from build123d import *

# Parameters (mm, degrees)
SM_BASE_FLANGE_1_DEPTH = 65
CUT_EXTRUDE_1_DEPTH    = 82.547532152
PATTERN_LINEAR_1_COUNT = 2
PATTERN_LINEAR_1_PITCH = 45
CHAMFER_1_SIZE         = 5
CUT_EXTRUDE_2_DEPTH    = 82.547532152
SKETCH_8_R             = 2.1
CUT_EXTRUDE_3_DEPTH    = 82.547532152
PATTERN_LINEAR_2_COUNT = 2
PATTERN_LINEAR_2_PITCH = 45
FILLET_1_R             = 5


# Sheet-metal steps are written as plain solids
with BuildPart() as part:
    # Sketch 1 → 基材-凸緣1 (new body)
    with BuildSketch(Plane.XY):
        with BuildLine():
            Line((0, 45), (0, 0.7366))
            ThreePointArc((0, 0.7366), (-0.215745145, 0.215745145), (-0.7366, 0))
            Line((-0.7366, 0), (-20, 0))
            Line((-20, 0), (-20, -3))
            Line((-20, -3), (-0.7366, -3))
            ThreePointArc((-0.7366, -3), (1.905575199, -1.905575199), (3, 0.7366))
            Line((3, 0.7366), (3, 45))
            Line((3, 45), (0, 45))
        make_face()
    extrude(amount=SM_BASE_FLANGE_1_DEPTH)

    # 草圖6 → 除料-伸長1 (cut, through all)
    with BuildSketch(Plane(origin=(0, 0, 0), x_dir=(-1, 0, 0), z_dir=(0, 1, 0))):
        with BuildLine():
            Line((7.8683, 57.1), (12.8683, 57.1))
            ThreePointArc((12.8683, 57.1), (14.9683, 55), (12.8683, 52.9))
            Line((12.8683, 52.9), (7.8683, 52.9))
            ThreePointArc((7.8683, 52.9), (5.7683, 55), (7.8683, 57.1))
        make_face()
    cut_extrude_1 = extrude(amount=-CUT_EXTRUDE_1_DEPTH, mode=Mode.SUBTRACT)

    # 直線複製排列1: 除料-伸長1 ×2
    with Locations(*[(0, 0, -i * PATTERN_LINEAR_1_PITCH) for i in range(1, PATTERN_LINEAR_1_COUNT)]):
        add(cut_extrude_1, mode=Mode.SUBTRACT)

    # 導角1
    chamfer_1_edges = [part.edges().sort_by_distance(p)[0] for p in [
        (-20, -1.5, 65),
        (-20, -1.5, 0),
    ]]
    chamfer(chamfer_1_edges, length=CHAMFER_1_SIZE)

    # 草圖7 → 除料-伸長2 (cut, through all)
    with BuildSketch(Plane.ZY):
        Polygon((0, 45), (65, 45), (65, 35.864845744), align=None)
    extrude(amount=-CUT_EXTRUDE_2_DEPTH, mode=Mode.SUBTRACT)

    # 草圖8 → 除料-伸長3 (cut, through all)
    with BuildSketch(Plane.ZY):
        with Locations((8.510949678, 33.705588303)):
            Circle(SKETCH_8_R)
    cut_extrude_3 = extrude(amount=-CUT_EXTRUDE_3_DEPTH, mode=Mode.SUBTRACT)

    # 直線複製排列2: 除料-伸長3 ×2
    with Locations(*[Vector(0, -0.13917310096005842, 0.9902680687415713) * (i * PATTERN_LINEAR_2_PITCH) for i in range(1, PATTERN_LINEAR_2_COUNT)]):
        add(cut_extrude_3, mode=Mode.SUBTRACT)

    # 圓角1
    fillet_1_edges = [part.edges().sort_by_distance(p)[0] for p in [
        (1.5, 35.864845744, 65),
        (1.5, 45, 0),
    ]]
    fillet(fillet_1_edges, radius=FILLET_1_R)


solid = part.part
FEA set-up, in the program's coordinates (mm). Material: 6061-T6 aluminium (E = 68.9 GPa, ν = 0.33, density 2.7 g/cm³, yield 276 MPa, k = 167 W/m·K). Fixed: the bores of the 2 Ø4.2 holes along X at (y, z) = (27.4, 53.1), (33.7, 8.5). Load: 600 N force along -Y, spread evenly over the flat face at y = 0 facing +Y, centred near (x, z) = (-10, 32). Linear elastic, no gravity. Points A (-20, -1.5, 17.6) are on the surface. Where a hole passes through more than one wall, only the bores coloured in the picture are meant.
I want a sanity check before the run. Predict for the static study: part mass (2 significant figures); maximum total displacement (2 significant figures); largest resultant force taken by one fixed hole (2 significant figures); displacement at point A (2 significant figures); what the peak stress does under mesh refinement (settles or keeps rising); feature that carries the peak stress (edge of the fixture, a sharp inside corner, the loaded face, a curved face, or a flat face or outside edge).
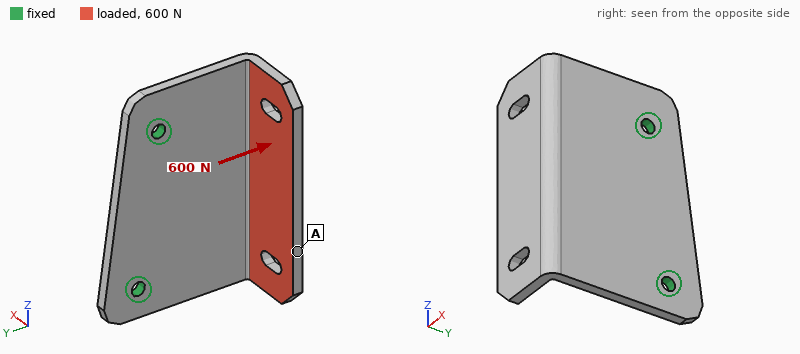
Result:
32 g
0.70 mm
320 N
0.66 mm
keeps rising
edge of the fixture
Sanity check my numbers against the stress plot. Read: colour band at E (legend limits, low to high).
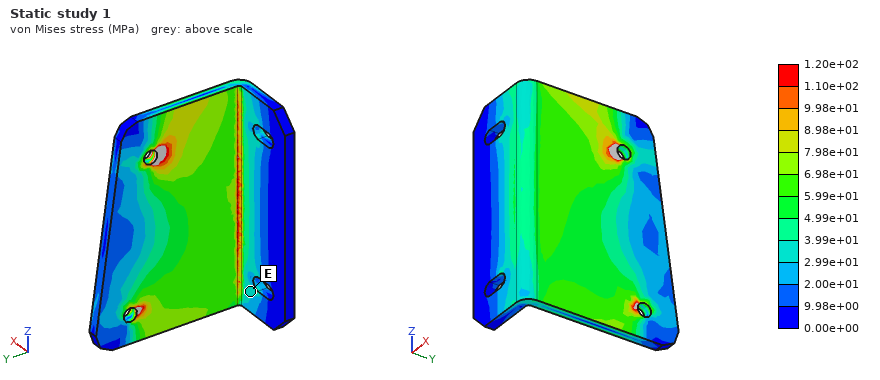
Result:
2.99e+01 to 3.99e+01 MPa
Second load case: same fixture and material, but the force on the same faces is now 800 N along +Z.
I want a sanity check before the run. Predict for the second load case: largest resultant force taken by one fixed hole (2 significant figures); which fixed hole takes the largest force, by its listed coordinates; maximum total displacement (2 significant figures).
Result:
730 N
(27.4, 53.1)
0.42 mm
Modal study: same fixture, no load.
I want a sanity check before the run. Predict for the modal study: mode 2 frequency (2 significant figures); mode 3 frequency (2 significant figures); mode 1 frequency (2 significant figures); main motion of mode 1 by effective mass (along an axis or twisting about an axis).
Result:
2000 Hz
3700 Hz
1100 Hz
along X
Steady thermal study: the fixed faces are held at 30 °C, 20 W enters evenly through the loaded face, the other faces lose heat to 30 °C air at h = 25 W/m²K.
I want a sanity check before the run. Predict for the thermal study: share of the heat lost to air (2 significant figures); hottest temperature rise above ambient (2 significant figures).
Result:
13 %
28 K
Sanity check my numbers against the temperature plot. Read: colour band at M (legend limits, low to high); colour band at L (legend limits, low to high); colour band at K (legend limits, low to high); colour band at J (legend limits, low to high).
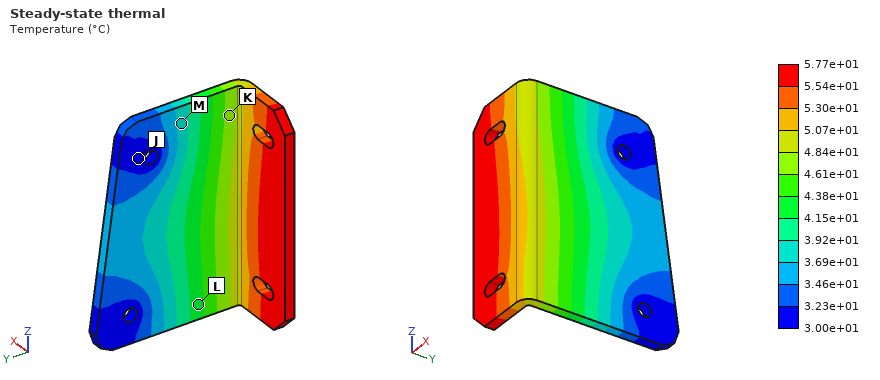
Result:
3.69e+01 to 3.92e+01 °C
4.15e+01 to 4.38e+01 °C
4.61e+01 to 4.84e+01 °C
3.00e+01 to 3.23e+01 °C
